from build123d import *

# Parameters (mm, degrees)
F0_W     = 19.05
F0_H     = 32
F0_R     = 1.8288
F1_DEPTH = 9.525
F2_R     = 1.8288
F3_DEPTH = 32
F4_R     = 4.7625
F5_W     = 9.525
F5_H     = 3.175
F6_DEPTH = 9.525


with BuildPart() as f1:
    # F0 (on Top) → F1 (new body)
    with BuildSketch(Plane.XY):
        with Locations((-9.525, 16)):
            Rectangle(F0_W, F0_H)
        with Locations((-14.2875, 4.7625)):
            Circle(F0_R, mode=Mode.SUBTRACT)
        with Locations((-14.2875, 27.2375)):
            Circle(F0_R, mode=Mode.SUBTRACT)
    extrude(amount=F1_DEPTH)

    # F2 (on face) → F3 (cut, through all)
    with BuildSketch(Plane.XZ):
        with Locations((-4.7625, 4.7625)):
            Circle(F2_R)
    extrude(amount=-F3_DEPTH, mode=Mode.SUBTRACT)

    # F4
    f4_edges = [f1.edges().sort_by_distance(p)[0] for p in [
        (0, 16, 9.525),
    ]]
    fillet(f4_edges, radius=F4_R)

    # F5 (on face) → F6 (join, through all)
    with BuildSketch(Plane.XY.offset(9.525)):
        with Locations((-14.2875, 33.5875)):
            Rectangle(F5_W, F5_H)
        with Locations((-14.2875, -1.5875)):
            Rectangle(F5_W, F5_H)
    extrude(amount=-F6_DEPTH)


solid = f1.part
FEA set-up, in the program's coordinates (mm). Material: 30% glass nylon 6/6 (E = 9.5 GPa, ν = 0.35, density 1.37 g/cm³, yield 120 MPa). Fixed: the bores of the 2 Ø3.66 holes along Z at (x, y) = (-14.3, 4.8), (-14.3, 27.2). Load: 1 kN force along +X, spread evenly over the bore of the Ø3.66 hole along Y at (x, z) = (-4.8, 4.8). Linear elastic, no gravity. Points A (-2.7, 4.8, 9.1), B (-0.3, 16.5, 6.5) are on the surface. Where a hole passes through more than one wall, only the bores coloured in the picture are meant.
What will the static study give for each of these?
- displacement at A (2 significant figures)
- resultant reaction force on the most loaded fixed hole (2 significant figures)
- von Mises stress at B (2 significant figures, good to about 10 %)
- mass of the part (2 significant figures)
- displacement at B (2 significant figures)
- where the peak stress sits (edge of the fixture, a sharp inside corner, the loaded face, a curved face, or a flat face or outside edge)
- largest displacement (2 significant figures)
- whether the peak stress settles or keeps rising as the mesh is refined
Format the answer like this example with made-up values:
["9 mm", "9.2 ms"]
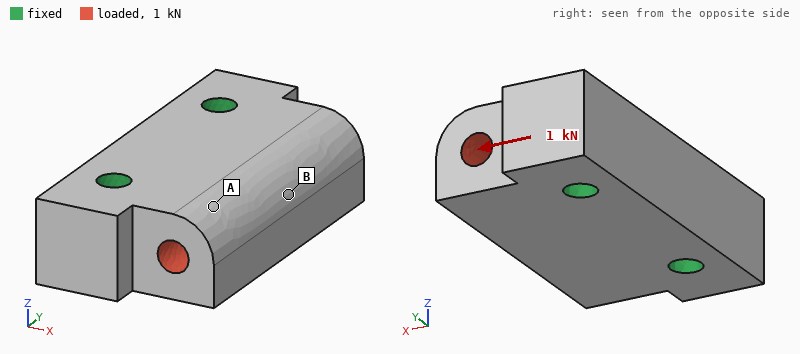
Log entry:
["3.9 µm", "510 N", "2.9 MPa", "7.8 g", "7.4 µm", "edge of the fixture", "8.3 µm", "keeps rising"]
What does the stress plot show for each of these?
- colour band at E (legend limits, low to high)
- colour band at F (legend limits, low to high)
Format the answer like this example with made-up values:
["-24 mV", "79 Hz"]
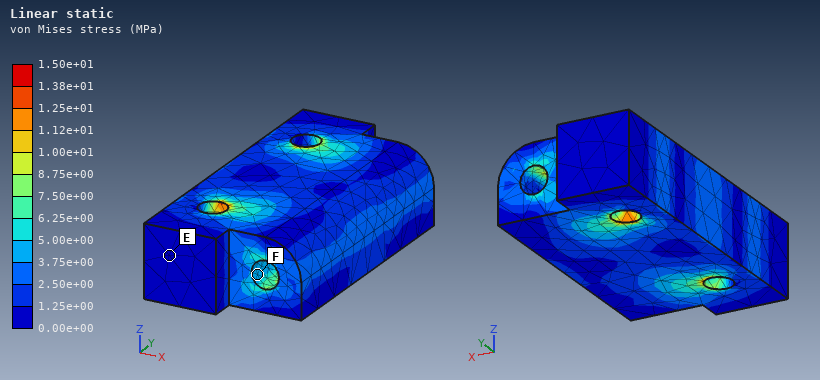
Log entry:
["0.00e+00 to 1.25e+00 MPa", "3.75e+00 to 5.00e+00 MPa"]
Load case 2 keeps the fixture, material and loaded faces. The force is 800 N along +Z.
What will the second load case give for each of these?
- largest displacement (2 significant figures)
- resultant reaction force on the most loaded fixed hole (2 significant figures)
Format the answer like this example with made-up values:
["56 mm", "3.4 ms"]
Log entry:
["44 µm", "400 N"]
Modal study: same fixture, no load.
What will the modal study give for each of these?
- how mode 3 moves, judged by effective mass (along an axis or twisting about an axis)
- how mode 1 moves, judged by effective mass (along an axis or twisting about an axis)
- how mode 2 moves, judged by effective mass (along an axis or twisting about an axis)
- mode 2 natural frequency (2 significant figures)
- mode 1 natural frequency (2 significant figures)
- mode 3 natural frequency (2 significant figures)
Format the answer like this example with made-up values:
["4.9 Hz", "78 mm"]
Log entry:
["along Y", "along Z", "twisting about X", "21 kHz", "14 kHz", "24 kHz"]
